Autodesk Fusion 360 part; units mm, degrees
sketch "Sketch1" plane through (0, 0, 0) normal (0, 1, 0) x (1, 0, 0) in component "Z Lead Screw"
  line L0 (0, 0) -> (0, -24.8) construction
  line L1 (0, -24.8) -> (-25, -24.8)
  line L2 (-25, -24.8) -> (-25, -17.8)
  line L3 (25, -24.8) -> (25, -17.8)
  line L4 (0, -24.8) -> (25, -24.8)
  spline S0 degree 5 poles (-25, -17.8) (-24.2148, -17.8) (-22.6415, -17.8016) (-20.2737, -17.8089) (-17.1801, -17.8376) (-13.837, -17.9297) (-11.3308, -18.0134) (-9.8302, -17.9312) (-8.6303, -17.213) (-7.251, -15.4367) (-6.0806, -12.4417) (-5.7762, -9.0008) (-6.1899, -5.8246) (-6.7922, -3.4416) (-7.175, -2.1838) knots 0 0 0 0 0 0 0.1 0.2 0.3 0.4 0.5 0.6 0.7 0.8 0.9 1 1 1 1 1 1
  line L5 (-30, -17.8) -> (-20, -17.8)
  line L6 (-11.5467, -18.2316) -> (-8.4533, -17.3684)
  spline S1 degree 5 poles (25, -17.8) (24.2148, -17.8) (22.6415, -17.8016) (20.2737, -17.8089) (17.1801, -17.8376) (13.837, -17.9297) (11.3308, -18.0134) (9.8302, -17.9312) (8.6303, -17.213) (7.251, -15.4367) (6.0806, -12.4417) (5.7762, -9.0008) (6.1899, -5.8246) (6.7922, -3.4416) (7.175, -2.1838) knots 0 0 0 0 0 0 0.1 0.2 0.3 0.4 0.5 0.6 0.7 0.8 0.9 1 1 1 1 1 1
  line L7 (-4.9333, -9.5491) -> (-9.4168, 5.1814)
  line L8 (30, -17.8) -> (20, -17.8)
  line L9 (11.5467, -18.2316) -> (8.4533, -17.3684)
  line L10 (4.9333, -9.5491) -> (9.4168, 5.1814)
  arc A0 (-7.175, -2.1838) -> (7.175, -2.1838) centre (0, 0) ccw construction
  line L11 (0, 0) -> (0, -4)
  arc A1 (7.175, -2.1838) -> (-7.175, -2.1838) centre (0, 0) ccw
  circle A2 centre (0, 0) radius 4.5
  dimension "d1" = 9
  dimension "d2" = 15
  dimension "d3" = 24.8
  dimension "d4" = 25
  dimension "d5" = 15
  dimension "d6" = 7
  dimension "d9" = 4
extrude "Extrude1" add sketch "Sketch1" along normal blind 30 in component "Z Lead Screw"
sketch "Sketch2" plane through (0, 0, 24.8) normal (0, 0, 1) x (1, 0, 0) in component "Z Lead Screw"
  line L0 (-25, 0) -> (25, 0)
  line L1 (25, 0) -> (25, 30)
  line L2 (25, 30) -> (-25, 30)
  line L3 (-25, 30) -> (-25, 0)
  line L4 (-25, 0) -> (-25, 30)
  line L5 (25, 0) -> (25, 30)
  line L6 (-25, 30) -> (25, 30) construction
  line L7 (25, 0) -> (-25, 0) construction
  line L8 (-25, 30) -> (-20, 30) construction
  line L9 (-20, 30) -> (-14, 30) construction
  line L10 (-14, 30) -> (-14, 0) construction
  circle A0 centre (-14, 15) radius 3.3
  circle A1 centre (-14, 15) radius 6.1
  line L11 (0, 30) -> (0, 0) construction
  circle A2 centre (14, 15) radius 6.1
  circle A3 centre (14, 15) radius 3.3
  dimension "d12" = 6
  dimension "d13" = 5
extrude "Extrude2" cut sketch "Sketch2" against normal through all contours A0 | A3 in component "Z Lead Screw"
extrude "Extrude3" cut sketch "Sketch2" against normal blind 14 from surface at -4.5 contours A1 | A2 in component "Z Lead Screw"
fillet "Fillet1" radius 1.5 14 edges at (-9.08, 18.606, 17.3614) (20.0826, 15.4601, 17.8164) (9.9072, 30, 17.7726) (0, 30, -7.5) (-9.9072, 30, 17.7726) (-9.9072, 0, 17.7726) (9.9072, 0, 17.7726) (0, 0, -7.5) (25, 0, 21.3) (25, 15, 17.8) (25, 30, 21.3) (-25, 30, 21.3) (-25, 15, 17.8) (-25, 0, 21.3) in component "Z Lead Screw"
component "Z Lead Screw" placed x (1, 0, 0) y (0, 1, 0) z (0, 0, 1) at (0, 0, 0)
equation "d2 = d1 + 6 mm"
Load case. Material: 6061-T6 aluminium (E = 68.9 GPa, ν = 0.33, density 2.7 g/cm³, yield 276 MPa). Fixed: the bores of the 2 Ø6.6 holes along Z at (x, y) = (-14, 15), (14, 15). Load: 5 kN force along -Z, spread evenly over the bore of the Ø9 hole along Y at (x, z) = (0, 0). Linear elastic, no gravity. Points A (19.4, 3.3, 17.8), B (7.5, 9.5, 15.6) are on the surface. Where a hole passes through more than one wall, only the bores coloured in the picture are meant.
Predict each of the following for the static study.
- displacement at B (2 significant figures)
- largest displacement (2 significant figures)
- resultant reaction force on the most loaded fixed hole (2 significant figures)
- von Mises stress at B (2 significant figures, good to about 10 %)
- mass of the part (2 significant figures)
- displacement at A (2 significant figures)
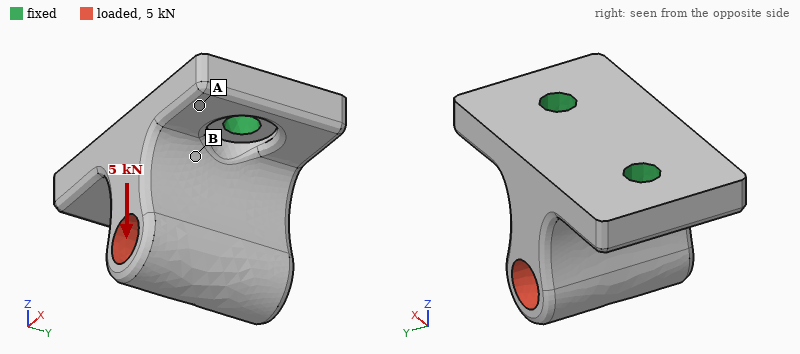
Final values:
10 µm
21 µm
2.7 kN
43 MPa
47 g
4.5 µm
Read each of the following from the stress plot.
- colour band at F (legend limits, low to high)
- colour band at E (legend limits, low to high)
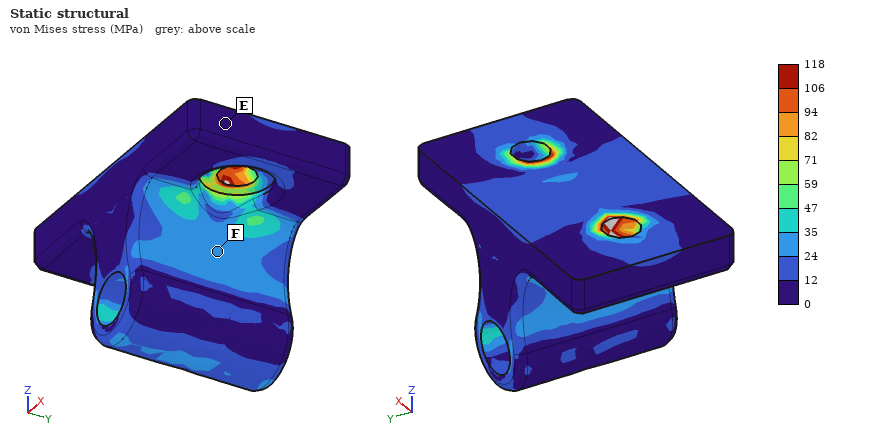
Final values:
24 to 35 MPa
0 to 12 MPa
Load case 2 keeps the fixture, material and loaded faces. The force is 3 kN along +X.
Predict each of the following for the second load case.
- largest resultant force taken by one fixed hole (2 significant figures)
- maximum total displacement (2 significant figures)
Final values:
3.2 kN
75 µm
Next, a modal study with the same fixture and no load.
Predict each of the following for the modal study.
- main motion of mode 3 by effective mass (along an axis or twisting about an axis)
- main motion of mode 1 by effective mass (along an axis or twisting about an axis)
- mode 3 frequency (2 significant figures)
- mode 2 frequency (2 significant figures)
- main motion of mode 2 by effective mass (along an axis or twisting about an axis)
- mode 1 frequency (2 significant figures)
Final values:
along Z
along Y
17 kHz
11 kHz
along X
6000 Hz
